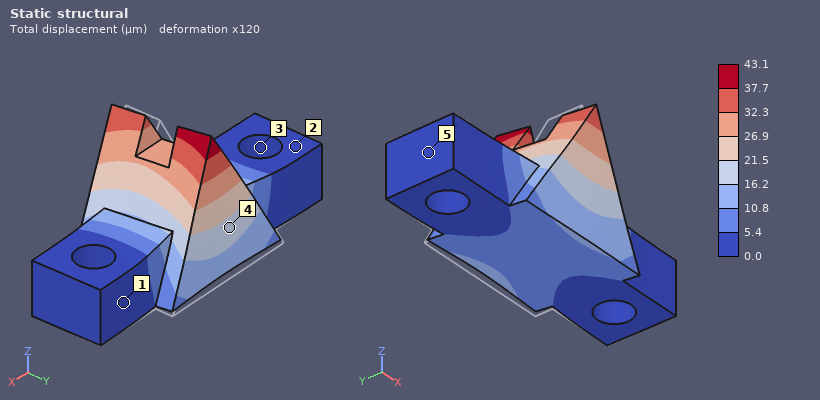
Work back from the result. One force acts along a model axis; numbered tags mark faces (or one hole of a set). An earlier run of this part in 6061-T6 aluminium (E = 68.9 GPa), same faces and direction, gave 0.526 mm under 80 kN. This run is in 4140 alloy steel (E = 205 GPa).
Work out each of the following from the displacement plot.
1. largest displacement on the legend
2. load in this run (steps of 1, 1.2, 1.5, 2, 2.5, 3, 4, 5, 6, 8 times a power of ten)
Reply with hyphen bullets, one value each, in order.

- 43.1 µm
- 20 kN
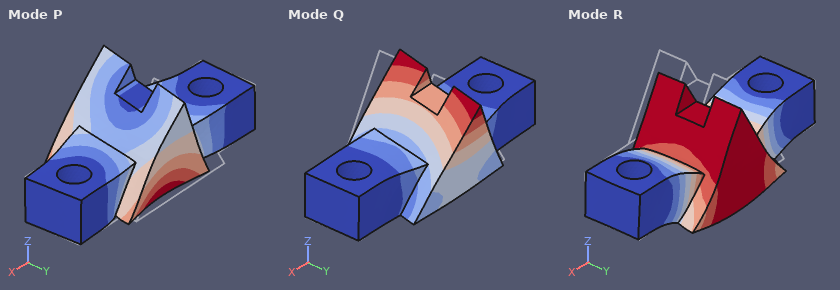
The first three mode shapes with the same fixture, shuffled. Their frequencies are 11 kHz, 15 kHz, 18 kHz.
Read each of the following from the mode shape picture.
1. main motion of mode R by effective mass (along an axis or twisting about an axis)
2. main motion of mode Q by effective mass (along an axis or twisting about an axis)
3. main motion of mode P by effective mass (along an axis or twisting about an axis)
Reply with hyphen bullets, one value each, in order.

- along Z
- along Y
- along Y
